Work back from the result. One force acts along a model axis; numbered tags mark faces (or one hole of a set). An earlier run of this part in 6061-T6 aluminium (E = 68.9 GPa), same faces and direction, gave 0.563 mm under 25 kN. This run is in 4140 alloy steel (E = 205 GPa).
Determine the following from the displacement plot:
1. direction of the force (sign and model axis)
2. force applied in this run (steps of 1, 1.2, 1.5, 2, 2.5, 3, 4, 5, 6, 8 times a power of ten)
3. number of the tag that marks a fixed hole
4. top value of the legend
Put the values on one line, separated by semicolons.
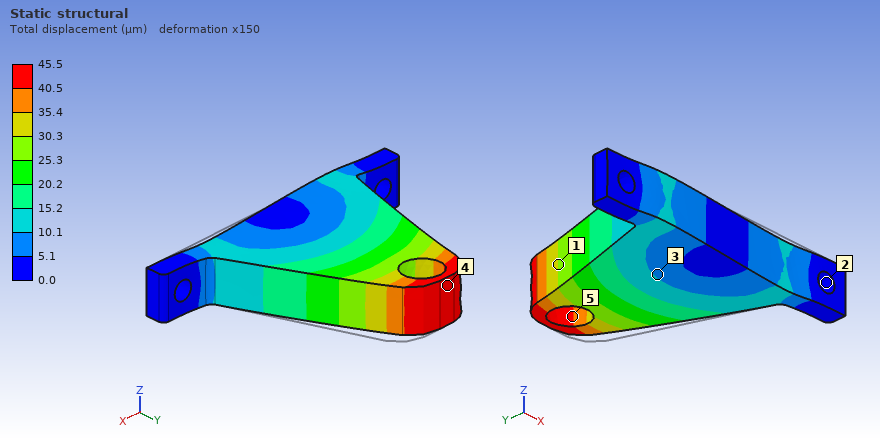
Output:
-X; 6 kN; 2; 45.5 µm
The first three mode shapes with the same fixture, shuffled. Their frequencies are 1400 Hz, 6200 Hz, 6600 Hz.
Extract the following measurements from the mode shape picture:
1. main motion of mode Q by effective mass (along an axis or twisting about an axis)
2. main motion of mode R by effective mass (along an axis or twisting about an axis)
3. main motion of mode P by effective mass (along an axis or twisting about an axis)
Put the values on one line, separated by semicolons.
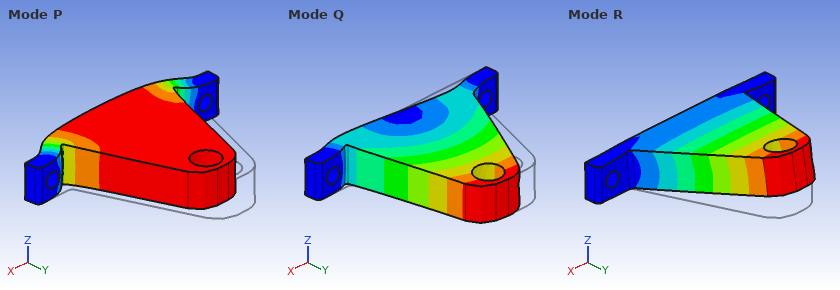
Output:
along X; along Z; along Y
